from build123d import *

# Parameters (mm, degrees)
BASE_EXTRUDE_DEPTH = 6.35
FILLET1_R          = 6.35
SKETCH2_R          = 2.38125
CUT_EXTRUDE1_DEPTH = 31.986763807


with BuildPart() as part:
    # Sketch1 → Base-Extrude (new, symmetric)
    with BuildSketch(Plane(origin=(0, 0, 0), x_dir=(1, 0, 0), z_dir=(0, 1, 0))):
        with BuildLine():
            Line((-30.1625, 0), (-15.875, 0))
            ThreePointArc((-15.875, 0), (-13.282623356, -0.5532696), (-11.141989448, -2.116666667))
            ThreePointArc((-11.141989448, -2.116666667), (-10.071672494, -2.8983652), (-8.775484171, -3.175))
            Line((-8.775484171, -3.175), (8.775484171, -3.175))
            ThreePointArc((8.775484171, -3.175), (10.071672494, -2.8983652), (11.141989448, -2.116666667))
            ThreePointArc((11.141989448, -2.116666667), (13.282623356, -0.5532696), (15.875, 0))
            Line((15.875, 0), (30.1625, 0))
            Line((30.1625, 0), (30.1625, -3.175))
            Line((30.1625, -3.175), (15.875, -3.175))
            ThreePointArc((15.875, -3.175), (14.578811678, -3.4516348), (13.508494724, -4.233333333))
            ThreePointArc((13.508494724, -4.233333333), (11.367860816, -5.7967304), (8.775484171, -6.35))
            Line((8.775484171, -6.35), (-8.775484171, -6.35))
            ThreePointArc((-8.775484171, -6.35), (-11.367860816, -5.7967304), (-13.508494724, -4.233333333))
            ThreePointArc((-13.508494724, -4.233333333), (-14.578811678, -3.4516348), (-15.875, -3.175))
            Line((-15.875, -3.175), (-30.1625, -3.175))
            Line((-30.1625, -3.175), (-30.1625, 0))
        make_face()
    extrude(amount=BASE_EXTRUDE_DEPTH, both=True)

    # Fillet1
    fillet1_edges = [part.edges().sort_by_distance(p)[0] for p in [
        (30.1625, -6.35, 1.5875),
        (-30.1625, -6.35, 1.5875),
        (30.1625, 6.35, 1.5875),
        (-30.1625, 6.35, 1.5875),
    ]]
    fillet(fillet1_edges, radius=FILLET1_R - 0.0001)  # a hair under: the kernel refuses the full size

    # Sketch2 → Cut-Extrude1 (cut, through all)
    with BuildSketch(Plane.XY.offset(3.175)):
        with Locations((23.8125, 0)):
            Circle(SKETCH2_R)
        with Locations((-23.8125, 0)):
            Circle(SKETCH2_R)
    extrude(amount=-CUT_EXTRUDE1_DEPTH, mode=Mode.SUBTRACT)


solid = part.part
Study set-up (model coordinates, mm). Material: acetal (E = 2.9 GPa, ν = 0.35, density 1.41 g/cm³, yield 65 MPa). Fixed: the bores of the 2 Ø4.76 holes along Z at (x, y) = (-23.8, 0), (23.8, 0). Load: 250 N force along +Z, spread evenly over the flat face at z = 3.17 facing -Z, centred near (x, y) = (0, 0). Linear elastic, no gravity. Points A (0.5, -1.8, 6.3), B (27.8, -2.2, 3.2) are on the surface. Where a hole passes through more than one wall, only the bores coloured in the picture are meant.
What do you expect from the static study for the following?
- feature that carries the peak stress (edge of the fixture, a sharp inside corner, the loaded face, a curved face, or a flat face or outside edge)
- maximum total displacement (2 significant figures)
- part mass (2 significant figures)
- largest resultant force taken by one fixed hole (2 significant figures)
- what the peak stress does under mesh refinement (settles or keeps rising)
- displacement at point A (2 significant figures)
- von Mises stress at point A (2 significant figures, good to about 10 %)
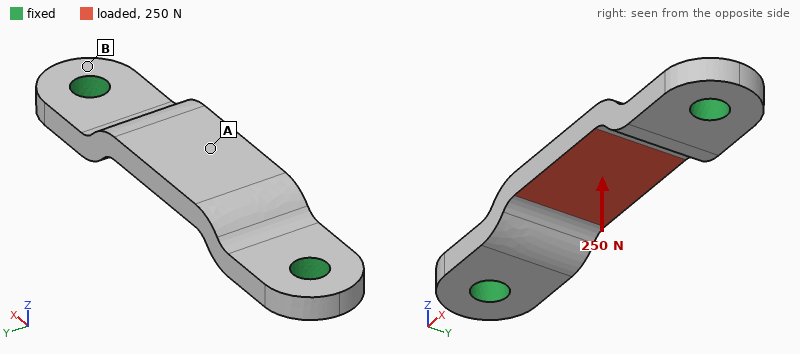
edge of the fixture
0.47 mm
3.2 g
350 N
keeps rising
0.44 mm
28 MPa
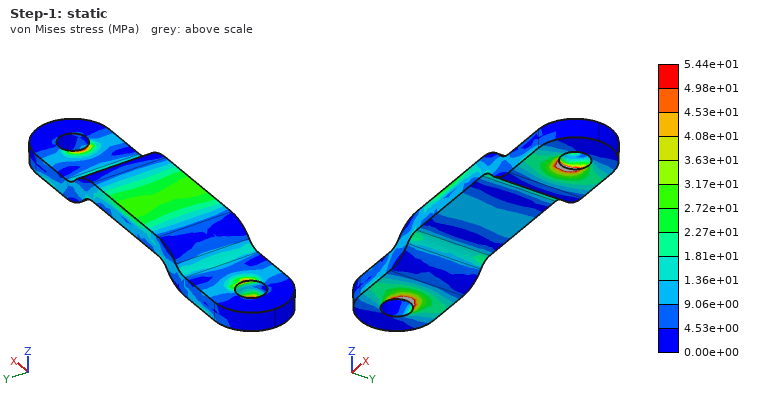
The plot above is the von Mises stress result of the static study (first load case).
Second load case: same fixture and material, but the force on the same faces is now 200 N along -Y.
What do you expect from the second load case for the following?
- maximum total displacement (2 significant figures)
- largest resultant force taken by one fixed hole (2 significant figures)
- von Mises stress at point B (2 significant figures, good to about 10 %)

0.18 mm
100 N
2.3 MPa
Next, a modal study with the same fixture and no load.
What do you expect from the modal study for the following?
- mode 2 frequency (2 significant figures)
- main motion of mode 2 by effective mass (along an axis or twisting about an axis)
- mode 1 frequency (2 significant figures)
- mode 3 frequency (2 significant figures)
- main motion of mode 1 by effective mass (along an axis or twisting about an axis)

3700 Hz
along Y
3400 Hz
5600 Hz
along Z
